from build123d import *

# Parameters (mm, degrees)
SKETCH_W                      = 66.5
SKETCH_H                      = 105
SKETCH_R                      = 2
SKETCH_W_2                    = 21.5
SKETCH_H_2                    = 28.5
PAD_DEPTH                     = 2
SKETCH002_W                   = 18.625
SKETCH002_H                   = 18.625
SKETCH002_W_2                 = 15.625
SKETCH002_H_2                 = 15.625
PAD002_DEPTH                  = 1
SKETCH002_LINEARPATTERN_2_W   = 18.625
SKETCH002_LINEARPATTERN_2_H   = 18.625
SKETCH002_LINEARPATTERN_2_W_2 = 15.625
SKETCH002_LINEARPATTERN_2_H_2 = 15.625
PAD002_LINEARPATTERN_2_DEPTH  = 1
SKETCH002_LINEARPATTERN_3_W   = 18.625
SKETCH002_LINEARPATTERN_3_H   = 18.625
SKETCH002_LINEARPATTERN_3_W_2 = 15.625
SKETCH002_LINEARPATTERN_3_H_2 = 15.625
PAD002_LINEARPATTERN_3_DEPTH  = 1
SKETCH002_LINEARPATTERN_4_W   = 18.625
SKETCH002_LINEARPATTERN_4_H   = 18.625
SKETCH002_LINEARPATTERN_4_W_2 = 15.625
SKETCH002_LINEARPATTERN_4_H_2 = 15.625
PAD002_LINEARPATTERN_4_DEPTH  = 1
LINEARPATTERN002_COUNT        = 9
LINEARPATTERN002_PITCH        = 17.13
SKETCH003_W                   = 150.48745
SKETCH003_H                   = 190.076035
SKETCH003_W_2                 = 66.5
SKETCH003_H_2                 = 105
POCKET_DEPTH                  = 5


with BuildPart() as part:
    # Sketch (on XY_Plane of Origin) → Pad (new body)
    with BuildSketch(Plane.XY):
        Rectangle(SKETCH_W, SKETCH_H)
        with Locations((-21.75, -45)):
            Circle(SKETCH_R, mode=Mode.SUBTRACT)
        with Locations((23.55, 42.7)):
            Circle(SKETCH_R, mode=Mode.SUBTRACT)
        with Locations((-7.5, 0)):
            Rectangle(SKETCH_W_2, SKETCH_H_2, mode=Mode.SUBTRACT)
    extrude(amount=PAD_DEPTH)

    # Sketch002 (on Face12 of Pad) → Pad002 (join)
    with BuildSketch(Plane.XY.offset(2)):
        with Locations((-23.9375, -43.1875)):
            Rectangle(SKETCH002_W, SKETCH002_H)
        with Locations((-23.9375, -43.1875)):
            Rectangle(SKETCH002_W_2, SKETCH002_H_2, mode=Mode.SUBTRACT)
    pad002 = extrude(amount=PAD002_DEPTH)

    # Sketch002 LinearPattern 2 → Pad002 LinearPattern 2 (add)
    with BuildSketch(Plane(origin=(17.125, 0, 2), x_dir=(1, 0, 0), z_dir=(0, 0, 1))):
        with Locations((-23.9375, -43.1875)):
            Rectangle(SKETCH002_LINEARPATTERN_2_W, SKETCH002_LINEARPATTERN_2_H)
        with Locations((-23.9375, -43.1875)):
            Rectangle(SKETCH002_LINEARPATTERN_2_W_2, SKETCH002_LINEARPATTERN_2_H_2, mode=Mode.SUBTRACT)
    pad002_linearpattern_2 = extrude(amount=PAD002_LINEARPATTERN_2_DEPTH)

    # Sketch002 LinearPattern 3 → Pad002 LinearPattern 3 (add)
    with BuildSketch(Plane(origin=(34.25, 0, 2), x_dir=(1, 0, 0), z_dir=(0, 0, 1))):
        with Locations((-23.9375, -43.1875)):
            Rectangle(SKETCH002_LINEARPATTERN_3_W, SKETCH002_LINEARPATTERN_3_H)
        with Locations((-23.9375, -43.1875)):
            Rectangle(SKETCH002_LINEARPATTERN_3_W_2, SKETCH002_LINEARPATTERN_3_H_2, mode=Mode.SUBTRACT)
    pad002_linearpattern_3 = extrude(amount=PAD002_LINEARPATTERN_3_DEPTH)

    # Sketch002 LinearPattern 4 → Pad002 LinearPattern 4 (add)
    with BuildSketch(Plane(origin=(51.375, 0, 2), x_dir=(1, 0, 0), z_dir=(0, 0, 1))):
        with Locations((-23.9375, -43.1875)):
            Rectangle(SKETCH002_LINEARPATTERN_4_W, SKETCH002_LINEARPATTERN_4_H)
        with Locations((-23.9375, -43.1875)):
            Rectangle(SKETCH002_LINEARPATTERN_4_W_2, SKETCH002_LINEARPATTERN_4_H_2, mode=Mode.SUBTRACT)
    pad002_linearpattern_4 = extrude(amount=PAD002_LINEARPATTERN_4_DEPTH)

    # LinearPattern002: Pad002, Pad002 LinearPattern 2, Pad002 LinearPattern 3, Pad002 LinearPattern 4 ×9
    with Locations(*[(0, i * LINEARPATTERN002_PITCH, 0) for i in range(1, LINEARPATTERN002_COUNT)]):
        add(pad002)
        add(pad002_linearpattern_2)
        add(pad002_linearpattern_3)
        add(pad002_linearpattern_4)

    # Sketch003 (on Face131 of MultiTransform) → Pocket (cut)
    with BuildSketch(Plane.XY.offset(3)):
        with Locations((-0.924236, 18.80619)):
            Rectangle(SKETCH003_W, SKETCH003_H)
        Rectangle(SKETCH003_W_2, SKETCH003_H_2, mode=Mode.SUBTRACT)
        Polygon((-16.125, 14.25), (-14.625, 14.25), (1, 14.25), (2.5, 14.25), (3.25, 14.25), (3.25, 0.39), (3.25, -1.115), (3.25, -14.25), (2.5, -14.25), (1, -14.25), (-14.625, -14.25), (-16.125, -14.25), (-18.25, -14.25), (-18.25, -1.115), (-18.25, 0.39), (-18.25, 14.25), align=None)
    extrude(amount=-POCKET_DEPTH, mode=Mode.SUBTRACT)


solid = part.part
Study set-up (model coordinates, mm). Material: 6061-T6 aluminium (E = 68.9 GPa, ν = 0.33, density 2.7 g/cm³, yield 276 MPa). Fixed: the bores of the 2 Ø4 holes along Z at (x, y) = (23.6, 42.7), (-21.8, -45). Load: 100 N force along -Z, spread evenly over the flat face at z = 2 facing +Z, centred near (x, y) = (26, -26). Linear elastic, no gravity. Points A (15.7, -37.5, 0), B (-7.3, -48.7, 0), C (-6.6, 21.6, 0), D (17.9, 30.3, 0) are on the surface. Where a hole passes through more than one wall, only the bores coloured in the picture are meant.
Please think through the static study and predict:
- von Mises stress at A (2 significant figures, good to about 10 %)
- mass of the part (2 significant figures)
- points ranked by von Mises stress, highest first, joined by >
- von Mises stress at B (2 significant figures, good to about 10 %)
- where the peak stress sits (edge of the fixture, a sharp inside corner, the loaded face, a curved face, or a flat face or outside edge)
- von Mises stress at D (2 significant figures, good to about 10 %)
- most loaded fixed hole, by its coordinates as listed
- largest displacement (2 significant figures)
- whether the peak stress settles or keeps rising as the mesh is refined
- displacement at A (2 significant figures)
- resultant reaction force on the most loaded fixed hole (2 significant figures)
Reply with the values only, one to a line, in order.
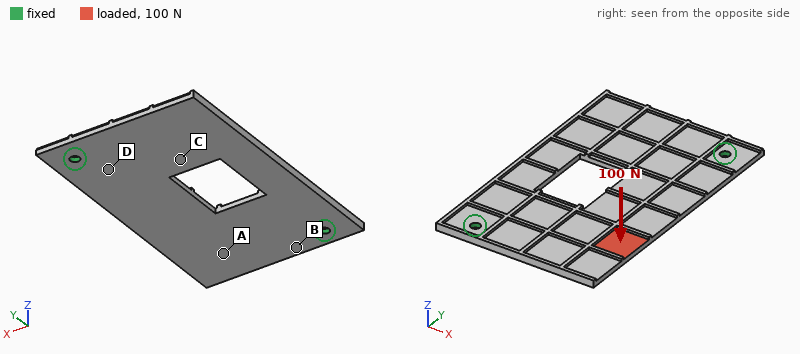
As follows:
24 MPa
37 g
B > D > A > C
64 MPa
edge of the fixture
47 MPa
(-21.8, -45)
1.2 mm
keeps rising
0.69 mm
64 N
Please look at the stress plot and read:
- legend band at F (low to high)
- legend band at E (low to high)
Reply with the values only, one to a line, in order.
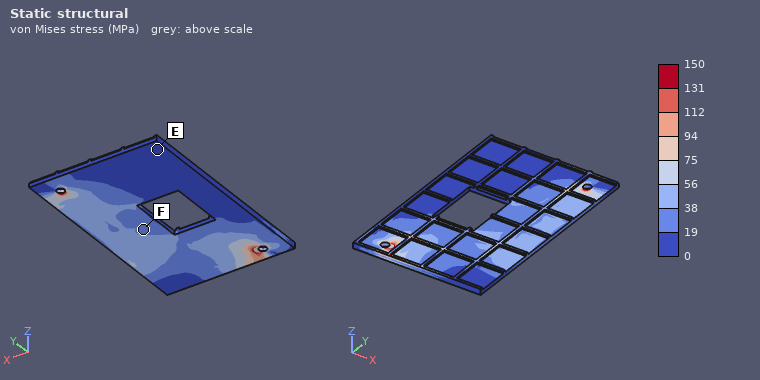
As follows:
19 to 38 MPa
0 to 19 MPa
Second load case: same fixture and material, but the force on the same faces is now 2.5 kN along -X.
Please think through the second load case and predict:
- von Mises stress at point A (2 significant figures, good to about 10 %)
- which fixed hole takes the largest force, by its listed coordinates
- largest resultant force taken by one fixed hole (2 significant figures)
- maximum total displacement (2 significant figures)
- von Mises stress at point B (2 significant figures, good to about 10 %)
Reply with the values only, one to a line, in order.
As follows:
38 MPa
(-21.8, -45)
2.1 kN
0.84 mm
9.3 MPa
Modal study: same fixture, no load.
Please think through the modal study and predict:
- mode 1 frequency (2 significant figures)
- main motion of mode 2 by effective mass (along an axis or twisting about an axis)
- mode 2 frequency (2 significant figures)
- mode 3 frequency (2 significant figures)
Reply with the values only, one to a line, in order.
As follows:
580 Hz
along Z
710 Hz
1300 Hz
